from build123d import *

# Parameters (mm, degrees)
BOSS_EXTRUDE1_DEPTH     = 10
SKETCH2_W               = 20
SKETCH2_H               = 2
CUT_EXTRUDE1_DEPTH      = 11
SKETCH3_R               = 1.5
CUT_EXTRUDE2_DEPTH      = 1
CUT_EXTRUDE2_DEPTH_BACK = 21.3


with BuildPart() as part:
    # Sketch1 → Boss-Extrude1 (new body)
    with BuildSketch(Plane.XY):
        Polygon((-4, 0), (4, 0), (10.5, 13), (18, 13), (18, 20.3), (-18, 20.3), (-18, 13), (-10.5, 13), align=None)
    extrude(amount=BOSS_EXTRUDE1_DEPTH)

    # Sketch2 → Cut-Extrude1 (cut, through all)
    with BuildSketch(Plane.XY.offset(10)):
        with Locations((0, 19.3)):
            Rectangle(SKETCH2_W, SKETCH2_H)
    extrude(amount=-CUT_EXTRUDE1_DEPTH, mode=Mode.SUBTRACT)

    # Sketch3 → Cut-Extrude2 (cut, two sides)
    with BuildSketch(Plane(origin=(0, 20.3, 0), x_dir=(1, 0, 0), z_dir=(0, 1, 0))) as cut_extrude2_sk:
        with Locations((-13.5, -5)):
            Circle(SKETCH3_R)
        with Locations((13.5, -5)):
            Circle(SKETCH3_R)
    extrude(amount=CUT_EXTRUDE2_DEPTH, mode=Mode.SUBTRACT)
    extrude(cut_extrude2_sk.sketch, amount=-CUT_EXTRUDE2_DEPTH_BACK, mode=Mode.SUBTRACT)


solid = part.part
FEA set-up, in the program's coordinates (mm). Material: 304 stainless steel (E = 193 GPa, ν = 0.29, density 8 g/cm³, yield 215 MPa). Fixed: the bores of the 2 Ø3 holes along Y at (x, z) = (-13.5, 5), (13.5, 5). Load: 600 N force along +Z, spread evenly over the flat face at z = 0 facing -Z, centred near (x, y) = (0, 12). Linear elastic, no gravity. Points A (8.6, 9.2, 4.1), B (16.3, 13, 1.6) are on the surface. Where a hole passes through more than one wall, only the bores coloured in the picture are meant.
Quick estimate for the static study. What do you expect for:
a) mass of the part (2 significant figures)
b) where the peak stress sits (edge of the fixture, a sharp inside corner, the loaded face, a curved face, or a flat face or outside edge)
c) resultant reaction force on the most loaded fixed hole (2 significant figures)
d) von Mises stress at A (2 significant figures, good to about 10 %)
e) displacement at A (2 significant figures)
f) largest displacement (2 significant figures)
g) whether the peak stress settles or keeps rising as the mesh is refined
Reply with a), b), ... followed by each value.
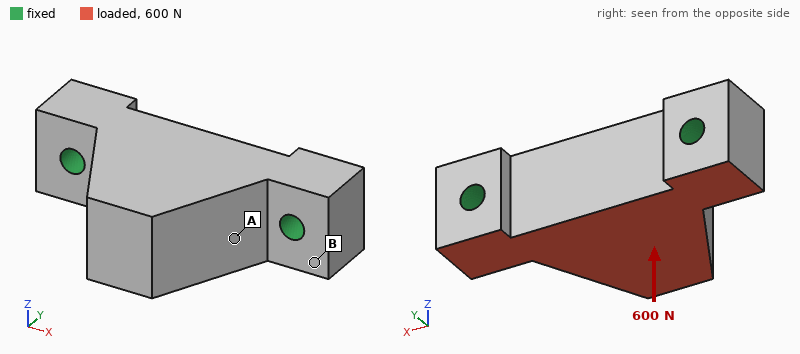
a) 32 g
b) edge of the fixture
c) 300 N
d) 9.7 MPa
e) 1.6 µm
f) 3.9 µm
g) keeps rising
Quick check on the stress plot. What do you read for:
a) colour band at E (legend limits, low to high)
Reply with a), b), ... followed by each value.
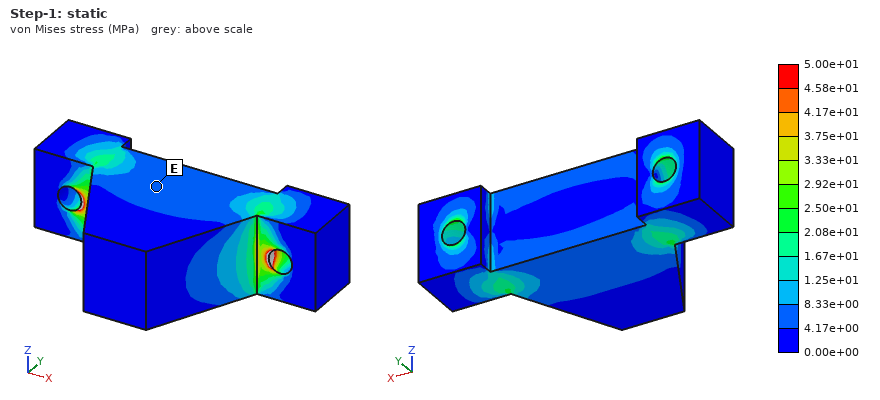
a) 4.17e+00 to 8.33e+00 MPa
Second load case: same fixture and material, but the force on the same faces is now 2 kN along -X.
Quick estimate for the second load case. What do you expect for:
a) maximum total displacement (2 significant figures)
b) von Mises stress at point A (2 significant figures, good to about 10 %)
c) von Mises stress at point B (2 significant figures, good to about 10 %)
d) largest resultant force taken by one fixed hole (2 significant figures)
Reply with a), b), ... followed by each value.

a) 2.5 µm
b) 14 MPa
c) 7.9 MPa
d) 1.1 kN
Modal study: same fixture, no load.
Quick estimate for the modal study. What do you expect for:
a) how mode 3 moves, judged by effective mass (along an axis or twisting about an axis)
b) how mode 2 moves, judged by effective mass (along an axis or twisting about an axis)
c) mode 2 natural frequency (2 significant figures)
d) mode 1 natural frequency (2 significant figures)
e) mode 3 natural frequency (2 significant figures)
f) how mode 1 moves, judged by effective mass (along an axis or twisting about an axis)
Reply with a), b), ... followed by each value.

a) along X
b) along Y
c) 32 kHz
d) 14 kHz
e) 37 kHz
f) along Z
